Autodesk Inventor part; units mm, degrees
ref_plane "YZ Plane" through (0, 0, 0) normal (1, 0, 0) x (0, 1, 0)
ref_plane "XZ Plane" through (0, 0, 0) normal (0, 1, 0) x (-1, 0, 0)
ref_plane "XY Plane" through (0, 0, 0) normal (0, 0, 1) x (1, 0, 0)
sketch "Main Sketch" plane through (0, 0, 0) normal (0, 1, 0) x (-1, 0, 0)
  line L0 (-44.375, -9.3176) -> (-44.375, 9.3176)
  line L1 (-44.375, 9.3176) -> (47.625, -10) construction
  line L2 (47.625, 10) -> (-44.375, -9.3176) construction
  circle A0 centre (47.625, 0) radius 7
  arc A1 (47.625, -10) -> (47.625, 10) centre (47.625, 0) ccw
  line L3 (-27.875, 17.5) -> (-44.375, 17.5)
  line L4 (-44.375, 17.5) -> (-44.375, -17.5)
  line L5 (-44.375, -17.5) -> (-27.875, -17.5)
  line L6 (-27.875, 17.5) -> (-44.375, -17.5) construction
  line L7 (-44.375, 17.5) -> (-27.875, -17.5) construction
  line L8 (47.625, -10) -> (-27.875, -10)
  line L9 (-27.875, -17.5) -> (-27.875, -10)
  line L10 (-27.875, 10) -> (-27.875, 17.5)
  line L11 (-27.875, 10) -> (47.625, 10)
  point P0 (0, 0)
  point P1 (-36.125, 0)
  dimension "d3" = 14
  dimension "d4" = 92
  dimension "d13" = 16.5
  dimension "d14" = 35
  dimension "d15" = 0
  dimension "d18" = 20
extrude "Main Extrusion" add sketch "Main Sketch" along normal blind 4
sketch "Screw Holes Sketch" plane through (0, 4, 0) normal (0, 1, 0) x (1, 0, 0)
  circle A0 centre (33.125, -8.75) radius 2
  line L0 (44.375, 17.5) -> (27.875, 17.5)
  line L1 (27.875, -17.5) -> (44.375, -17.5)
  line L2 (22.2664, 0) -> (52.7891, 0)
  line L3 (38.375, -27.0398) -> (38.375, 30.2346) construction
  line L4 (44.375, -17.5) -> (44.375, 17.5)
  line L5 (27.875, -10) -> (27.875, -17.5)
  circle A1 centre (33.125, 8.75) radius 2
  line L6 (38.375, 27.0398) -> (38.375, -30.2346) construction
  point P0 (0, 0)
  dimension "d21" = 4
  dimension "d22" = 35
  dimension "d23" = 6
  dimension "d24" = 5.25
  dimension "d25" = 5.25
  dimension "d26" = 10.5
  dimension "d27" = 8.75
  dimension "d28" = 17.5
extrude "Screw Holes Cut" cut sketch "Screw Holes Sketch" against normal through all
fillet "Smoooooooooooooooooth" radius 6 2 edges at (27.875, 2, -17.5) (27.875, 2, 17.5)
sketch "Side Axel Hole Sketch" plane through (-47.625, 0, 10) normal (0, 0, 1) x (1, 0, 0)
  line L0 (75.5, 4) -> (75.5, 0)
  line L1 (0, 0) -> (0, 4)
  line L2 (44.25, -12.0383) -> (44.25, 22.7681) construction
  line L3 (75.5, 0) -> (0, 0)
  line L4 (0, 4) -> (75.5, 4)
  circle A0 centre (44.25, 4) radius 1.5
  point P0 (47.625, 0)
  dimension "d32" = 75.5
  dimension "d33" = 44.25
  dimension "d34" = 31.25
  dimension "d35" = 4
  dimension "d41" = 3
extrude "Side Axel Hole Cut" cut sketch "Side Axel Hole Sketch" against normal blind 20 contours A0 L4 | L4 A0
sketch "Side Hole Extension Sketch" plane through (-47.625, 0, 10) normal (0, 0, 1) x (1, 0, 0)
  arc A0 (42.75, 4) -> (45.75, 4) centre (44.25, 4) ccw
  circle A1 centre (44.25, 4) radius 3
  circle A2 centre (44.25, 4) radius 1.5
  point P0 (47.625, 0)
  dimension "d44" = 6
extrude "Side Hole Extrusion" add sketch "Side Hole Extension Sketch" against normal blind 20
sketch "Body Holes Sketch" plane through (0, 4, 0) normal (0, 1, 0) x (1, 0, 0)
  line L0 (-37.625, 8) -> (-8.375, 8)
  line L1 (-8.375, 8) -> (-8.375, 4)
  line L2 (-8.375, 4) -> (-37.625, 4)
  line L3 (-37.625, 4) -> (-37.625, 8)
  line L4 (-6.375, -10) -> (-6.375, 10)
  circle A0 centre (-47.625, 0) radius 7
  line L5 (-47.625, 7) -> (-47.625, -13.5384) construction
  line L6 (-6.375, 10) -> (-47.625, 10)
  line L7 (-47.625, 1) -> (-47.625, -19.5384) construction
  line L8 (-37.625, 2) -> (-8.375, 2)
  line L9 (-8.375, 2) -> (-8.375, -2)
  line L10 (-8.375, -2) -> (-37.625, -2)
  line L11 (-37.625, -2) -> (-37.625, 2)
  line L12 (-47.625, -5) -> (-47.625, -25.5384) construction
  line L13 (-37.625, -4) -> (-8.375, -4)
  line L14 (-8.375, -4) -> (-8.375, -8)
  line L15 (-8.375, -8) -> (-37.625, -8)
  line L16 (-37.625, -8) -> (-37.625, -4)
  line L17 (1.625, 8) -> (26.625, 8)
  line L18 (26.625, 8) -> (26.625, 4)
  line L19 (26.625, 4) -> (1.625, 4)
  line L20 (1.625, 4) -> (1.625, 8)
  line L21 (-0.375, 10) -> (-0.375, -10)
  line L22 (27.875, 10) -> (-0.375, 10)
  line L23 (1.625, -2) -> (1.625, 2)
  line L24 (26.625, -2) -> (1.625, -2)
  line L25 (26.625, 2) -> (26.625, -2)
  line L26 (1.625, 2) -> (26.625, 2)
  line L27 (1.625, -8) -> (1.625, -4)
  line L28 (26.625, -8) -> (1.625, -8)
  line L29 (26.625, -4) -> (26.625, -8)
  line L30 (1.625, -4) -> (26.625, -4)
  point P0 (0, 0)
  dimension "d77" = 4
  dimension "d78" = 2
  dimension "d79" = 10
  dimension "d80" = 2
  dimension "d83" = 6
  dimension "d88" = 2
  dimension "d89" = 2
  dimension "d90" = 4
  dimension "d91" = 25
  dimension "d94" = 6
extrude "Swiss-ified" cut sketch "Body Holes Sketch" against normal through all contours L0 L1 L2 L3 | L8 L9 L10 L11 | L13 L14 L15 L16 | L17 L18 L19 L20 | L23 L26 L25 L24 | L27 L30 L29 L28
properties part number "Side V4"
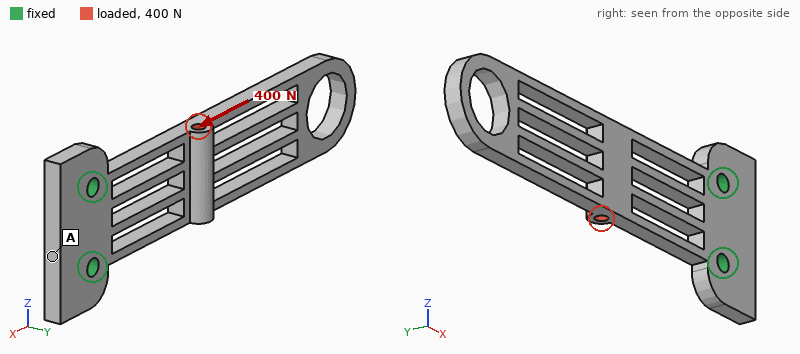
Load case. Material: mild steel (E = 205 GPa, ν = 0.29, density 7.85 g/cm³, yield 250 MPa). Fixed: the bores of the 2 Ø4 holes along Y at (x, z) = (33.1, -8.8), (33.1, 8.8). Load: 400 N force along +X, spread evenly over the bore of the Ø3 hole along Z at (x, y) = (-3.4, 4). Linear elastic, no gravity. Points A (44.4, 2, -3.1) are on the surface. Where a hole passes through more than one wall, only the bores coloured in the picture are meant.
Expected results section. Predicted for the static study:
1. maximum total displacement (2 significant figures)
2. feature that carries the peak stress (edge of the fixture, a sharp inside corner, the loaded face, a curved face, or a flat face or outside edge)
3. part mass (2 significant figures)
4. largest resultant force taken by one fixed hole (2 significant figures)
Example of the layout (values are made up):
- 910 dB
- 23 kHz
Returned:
- 0.20 mm
- a flat face or outside edge
- 45 g
- 200 N
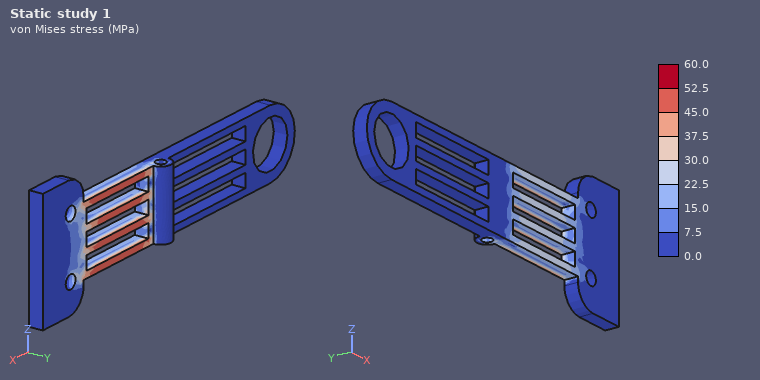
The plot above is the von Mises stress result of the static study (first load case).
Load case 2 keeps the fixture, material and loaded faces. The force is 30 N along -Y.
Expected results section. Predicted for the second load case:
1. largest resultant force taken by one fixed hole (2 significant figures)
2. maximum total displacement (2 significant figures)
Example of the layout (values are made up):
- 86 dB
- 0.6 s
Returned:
- 15 N
- 0.14 mm
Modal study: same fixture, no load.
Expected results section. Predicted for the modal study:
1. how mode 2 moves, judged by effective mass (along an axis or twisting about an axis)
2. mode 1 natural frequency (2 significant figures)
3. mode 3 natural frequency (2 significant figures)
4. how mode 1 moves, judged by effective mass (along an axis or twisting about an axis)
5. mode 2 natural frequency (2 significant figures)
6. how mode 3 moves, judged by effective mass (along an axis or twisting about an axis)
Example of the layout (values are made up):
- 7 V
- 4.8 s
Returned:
- along Z
- 410 Hz
- 2100 Hz
- along Y
- 960 Hz
- twisting about X
